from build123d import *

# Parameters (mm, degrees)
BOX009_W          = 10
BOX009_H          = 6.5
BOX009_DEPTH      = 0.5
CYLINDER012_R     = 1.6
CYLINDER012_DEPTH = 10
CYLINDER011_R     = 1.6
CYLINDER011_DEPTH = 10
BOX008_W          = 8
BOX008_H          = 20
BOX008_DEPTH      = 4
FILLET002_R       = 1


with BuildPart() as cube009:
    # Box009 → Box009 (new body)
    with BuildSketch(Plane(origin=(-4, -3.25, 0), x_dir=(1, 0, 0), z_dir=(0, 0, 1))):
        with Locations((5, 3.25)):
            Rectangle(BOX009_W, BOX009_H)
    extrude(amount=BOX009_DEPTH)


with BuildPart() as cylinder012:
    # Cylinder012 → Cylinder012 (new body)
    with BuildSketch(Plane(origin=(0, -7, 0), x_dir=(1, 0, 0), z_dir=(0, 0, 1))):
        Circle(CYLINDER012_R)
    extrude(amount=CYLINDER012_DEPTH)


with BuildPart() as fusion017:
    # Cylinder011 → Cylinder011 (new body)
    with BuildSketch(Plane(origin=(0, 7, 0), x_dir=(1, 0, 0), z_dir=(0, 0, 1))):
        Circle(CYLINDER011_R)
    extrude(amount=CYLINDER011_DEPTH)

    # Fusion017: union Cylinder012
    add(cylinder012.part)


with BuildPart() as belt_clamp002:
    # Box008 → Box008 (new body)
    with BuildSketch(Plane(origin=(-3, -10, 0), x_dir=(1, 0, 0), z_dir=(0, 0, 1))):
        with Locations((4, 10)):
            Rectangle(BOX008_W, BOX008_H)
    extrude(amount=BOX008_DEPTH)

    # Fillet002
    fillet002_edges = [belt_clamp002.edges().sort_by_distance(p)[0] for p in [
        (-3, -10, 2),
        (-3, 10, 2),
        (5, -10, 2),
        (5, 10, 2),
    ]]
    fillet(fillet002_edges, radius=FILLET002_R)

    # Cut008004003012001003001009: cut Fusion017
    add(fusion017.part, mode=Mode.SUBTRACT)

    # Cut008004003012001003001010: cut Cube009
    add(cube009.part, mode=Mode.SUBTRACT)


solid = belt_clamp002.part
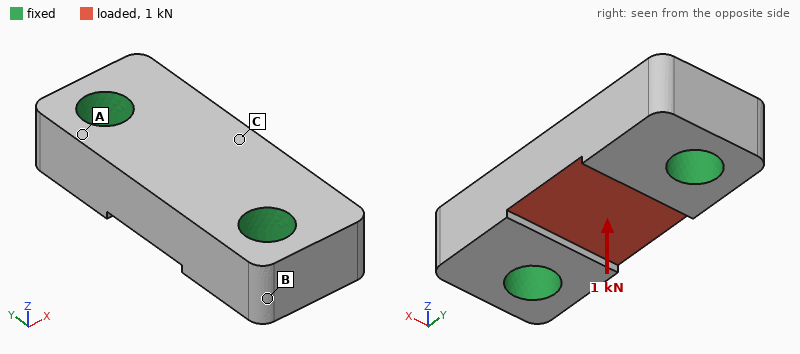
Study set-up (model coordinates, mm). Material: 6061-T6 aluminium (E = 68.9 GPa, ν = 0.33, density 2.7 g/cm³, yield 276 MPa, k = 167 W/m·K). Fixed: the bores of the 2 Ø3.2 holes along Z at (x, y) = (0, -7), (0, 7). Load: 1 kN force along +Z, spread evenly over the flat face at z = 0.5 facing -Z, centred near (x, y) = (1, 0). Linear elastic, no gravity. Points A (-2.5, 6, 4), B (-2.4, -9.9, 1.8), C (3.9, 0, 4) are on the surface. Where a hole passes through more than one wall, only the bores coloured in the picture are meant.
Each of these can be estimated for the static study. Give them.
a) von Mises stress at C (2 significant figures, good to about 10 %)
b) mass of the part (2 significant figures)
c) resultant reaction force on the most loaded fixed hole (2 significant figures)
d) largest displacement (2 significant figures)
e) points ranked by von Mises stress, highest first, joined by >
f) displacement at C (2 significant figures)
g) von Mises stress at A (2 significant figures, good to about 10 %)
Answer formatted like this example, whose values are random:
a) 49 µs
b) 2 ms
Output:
a) 54 MPa
b) 1.5 g
c) 500 N
d) 9.4 µm
e) C > A > B
f) 7.9 µm
g) 32 MPa
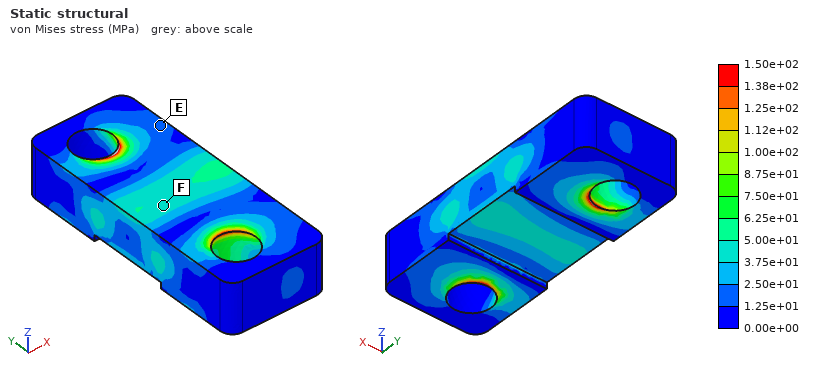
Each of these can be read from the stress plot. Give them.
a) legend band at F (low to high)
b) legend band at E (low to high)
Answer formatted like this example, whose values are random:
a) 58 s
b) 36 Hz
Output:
a) 3.75e+01 to 5.00e+01 MPa
b) 1.25e+01 to 2.50e+01 MPa
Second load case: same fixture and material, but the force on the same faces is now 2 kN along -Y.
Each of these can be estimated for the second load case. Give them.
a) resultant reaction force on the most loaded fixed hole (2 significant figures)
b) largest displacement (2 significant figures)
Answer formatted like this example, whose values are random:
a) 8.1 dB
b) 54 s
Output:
a) 1.0 kN
b) 5.2 µm
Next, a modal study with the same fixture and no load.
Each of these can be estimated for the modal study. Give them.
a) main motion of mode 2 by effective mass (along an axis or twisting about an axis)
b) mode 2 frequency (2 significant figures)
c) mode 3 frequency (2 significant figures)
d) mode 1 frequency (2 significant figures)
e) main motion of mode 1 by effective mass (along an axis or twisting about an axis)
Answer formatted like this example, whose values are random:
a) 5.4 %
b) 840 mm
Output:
a) along X
b) 99 kHz
c) 100 kHz
d) 79 kHz
e) along Z
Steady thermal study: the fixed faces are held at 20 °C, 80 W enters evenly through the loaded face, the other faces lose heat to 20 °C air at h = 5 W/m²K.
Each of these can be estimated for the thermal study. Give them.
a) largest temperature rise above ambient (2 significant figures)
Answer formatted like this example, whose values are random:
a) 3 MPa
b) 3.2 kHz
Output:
a) 49 K
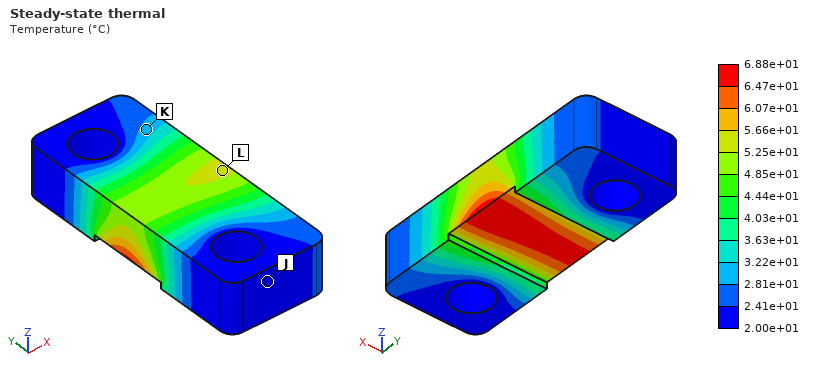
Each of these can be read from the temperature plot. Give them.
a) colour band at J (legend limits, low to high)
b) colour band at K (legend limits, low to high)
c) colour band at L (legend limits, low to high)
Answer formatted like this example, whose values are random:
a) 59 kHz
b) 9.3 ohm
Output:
a) 2.00e+01 to 2.41e+01 °C
b) 2.81e+01 to 3.22e+01 °C
c) 5.25e+01 to 5.66e+01 °C
